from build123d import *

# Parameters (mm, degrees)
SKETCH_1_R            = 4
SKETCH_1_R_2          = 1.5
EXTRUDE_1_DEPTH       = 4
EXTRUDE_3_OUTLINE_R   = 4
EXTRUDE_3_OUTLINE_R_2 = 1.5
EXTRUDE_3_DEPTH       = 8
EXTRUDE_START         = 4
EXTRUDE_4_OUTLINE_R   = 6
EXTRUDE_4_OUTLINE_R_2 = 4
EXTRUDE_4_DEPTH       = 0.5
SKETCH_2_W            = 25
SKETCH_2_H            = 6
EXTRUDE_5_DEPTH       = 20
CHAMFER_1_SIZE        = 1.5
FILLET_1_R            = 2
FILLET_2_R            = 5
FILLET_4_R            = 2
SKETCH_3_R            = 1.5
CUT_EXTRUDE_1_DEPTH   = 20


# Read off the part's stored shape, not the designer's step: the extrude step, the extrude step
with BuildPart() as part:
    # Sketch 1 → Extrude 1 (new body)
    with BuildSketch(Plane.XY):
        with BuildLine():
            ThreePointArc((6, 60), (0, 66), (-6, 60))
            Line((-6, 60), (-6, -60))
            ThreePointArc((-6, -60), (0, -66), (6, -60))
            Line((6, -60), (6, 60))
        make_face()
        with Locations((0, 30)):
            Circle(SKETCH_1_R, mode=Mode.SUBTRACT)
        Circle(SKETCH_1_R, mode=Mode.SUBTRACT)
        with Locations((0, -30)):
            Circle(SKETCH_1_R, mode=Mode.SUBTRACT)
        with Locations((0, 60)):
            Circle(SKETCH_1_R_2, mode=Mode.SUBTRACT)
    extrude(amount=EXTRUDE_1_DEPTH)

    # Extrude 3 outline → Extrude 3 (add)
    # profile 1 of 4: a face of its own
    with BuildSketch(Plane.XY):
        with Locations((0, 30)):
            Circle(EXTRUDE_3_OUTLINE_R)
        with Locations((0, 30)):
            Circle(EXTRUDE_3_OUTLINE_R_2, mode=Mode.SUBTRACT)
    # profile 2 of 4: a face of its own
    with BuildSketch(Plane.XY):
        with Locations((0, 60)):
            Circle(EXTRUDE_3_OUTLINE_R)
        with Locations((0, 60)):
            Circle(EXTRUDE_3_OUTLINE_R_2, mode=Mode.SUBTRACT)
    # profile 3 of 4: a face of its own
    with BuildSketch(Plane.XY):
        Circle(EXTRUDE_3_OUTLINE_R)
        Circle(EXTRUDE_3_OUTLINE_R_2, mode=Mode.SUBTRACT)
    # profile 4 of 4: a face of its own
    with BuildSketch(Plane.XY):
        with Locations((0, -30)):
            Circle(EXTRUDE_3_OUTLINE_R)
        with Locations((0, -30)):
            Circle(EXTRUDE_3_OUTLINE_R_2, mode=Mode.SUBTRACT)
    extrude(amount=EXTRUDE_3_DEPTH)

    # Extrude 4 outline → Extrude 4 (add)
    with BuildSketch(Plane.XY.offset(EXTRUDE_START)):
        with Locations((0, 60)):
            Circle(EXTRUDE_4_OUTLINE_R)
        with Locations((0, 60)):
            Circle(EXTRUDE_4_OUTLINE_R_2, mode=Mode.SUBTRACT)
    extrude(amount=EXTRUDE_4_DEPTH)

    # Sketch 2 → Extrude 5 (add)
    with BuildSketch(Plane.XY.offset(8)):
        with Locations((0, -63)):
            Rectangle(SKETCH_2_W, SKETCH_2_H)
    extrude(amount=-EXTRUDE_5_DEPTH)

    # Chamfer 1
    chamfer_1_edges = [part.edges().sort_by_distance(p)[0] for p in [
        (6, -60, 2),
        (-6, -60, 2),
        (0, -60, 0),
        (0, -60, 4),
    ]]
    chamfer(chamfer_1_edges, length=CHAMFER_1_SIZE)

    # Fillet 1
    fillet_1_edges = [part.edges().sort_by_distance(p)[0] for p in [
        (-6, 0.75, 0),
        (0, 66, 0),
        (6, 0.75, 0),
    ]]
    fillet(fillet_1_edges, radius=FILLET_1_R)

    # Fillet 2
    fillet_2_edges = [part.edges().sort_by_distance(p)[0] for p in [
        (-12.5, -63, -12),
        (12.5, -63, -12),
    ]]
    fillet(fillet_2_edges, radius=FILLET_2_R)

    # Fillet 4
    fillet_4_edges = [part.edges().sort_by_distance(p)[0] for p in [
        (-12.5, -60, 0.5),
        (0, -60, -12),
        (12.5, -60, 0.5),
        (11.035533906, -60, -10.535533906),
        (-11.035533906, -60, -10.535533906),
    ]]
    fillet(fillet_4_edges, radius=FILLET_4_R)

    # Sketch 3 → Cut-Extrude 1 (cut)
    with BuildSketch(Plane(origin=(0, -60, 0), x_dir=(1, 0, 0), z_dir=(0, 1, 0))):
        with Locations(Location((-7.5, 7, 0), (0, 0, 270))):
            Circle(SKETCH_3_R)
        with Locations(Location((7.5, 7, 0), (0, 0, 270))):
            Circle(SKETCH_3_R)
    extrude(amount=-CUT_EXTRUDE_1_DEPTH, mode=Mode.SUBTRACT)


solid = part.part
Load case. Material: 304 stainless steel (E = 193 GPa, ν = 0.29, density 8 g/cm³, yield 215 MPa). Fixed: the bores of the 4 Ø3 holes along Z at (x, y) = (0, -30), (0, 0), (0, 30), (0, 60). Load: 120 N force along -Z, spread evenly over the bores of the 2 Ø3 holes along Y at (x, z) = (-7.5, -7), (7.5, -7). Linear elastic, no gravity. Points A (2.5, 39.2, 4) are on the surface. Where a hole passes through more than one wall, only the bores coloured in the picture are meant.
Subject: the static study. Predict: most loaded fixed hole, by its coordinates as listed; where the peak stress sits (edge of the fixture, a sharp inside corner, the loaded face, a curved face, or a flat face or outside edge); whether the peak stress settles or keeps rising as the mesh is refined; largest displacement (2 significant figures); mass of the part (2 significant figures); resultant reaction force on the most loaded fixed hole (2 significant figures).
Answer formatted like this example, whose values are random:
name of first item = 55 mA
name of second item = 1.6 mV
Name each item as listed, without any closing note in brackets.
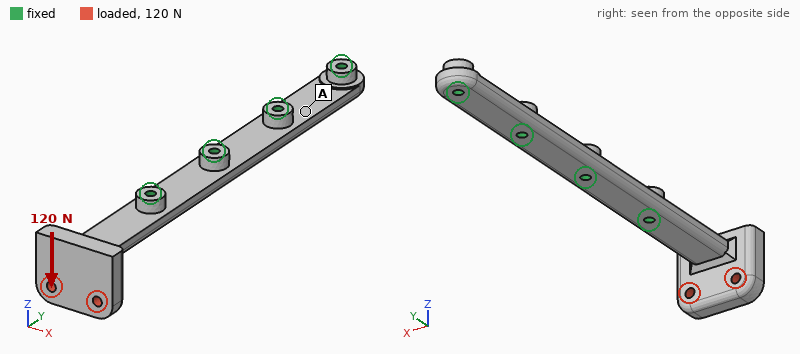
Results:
most loaded fixed hole, by its coordinates as listed = (0, -30)
where the peak stress sits = edge of the fixture
whether the peak stress settles or keeps rising as the mesh is refined = keeps rising
largest displacement = 0.14 mm
mass of the part = 74 g
resultant reaction force on the most loaded fixed hole = 120 N
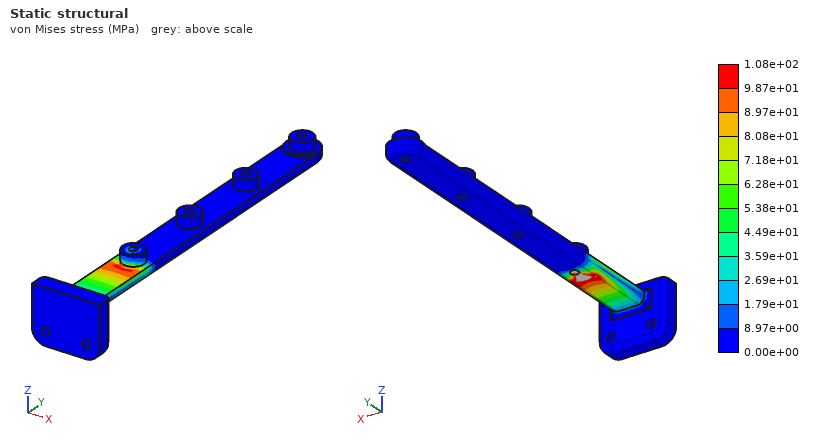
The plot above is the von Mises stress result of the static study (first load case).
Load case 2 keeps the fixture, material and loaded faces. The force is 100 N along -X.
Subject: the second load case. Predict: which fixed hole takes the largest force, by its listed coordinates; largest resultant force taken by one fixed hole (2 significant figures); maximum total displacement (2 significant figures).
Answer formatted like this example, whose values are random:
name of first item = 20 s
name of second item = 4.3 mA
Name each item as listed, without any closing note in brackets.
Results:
which fixed hole takes the largest force, by its listed coordinates = (0, -30)
largest resultant force taken by one fixed hole = 150 N
maximum total displacement = 43 µm
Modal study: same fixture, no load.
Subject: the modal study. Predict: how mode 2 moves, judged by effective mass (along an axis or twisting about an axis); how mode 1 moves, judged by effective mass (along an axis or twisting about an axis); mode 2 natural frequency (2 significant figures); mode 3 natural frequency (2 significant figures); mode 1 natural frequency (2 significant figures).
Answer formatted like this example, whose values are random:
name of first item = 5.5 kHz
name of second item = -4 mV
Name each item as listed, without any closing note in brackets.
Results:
how mode 2 moves, judged by effective mass = along X
how mode 1 moves, judged by effective mass = along Z
mode 2 natural frequency = 2100 Hz
mode 3 natural frequency = 3000 Hz
mode 1 natural frequency = 1000 Hz
